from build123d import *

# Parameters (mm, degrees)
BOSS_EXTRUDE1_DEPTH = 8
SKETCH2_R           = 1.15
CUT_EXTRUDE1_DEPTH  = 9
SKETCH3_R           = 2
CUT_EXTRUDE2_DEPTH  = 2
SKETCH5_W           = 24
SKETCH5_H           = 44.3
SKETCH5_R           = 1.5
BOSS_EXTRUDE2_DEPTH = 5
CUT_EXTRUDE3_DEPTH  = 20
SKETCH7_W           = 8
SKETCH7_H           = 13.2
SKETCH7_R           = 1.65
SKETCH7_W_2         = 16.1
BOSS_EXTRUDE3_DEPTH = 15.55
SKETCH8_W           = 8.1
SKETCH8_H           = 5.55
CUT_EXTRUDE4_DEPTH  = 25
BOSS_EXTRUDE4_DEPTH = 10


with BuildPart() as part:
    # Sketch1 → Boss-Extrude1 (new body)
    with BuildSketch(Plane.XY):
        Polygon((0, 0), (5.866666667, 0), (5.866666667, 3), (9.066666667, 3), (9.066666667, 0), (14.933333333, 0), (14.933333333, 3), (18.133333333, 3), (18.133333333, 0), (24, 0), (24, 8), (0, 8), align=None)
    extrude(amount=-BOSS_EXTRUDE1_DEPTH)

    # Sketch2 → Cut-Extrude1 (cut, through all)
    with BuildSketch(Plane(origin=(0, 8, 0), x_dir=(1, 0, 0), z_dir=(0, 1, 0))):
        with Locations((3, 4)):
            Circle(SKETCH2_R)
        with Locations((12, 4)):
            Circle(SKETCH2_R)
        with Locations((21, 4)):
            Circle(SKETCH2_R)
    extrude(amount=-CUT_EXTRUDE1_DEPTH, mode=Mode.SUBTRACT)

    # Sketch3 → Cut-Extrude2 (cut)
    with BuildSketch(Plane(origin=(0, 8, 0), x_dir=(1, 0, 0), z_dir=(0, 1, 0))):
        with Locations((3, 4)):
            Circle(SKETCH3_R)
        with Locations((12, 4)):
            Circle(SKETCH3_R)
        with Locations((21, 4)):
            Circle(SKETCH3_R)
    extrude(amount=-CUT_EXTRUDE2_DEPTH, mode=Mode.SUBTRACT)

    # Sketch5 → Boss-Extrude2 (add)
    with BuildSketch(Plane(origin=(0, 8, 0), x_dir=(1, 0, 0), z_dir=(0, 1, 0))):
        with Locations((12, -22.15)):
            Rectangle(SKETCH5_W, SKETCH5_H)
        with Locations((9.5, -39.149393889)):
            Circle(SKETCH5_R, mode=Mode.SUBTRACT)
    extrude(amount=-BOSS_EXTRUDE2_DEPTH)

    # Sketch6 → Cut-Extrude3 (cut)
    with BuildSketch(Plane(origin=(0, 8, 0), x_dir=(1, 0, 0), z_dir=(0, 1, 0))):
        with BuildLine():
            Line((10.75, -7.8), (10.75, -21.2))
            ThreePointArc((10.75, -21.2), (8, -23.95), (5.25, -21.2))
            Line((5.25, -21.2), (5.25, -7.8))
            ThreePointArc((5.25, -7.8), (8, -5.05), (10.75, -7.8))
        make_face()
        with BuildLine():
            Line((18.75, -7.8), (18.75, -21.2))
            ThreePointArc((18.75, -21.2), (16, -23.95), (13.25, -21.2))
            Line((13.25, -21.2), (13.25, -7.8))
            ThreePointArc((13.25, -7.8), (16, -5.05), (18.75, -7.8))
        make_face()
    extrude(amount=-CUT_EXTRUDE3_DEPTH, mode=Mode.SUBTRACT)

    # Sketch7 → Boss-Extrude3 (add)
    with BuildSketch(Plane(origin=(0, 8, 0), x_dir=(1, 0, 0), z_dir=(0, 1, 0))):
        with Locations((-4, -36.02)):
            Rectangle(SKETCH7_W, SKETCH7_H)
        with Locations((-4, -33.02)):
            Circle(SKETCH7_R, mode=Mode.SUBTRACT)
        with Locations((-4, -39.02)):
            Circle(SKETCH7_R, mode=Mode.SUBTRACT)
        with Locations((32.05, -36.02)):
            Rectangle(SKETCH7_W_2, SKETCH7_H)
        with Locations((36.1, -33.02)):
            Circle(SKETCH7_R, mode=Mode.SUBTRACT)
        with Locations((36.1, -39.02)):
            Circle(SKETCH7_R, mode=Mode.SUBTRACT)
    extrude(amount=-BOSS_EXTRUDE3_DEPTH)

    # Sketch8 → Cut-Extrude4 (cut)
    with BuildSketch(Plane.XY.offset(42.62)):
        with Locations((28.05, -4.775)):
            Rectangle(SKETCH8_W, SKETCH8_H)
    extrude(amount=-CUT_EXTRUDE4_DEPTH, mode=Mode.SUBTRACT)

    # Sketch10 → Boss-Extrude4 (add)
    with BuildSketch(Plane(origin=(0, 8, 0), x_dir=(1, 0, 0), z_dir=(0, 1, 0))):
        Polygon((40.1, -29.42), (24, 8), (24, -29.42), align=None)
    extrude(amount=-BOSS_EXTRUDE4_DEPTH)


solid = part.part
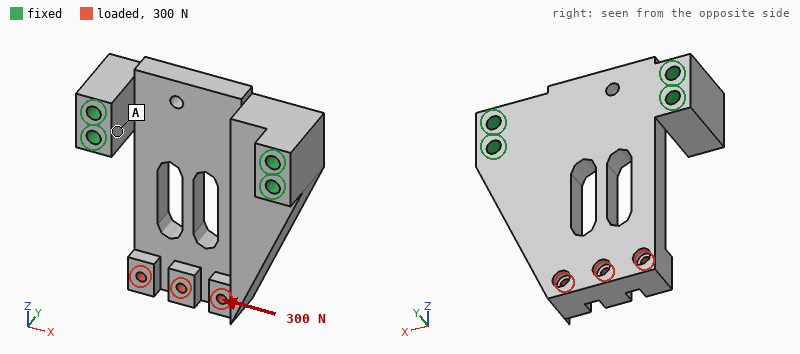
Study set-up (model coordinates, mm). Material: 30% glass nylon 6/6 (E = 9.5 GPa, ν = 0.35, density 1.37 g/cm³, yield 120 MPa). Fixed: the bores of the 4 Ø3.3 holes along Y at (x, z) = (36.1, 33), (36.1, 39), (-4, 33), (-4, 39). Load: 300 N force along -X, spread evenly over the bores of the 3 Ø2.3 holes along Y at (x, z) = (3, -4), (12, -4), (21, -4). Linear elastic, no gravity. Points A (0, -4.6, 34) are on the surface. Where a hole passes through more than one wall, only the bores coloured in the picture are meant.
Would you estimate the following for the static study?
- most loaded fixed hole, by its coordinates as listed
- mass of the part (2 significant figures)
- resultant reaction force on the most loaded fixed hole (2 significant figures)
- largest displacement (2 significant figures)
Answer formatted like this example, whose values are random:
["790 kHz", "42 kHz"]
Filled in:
["(36.1, 33)", "17 g", "420 N", "0.12 mm"]
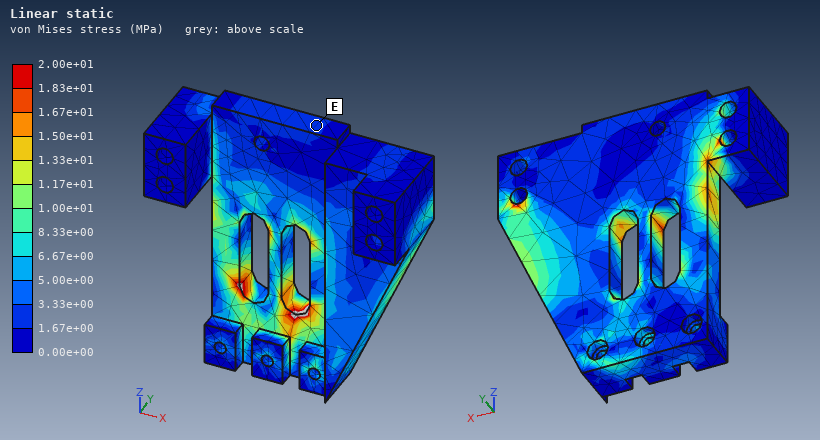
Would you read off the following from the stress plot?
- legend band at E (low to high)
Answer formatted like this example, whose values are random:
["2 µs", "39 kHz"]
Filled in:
["1.67e+00 to 3.33e+00 MPa"]
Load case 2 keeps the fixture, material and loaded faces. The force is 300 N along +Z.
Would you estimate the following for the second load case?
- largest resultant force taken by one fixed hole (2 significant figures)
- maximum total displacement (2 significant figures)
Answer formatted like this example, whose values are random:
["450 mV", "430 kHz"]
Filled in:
["110 N", "0.10 mm"]
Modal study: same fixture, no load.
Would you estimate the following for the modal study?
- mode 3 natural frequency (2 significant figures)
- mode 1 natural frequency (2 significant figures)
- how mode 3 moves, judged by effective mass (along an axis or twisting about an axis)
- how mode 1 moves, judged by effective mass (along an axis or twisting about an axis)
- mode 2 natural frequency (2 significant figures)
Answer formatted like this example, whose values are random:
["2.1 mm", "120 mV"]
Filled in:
["5300 Hz", "1800 Hz", "along X", "along Y", "4300 Hz"]
